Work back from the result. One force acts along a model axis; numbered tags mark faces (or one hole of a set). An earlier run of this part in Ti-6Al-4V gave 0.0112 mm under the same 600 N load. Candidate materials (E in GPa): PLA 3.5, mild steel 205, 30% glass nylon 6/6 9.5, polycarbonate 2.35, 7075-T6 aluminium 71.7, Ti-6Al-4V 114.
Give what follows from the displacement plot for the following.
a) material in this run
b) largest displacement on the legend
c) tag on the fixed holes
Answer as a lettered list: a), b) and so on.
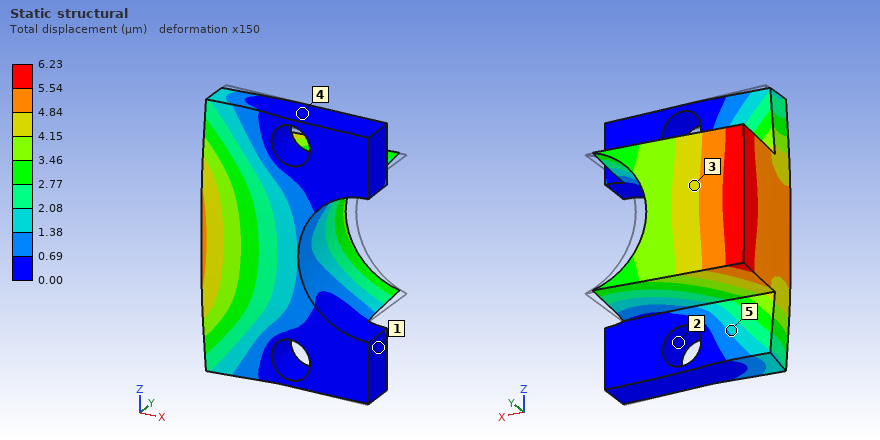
a) mild steel
b) 6.23 µm
c) 2
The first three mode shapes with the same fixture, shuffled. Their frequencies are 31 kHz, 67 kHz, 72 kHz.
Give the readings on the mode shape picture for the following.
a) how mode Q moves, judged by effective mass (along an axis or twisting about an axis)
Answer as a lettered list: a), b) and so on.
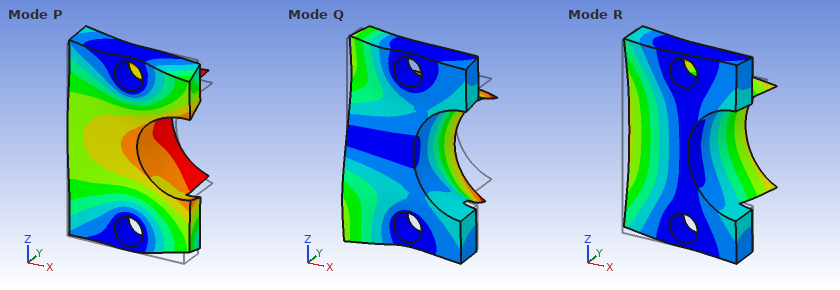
a) along Z
